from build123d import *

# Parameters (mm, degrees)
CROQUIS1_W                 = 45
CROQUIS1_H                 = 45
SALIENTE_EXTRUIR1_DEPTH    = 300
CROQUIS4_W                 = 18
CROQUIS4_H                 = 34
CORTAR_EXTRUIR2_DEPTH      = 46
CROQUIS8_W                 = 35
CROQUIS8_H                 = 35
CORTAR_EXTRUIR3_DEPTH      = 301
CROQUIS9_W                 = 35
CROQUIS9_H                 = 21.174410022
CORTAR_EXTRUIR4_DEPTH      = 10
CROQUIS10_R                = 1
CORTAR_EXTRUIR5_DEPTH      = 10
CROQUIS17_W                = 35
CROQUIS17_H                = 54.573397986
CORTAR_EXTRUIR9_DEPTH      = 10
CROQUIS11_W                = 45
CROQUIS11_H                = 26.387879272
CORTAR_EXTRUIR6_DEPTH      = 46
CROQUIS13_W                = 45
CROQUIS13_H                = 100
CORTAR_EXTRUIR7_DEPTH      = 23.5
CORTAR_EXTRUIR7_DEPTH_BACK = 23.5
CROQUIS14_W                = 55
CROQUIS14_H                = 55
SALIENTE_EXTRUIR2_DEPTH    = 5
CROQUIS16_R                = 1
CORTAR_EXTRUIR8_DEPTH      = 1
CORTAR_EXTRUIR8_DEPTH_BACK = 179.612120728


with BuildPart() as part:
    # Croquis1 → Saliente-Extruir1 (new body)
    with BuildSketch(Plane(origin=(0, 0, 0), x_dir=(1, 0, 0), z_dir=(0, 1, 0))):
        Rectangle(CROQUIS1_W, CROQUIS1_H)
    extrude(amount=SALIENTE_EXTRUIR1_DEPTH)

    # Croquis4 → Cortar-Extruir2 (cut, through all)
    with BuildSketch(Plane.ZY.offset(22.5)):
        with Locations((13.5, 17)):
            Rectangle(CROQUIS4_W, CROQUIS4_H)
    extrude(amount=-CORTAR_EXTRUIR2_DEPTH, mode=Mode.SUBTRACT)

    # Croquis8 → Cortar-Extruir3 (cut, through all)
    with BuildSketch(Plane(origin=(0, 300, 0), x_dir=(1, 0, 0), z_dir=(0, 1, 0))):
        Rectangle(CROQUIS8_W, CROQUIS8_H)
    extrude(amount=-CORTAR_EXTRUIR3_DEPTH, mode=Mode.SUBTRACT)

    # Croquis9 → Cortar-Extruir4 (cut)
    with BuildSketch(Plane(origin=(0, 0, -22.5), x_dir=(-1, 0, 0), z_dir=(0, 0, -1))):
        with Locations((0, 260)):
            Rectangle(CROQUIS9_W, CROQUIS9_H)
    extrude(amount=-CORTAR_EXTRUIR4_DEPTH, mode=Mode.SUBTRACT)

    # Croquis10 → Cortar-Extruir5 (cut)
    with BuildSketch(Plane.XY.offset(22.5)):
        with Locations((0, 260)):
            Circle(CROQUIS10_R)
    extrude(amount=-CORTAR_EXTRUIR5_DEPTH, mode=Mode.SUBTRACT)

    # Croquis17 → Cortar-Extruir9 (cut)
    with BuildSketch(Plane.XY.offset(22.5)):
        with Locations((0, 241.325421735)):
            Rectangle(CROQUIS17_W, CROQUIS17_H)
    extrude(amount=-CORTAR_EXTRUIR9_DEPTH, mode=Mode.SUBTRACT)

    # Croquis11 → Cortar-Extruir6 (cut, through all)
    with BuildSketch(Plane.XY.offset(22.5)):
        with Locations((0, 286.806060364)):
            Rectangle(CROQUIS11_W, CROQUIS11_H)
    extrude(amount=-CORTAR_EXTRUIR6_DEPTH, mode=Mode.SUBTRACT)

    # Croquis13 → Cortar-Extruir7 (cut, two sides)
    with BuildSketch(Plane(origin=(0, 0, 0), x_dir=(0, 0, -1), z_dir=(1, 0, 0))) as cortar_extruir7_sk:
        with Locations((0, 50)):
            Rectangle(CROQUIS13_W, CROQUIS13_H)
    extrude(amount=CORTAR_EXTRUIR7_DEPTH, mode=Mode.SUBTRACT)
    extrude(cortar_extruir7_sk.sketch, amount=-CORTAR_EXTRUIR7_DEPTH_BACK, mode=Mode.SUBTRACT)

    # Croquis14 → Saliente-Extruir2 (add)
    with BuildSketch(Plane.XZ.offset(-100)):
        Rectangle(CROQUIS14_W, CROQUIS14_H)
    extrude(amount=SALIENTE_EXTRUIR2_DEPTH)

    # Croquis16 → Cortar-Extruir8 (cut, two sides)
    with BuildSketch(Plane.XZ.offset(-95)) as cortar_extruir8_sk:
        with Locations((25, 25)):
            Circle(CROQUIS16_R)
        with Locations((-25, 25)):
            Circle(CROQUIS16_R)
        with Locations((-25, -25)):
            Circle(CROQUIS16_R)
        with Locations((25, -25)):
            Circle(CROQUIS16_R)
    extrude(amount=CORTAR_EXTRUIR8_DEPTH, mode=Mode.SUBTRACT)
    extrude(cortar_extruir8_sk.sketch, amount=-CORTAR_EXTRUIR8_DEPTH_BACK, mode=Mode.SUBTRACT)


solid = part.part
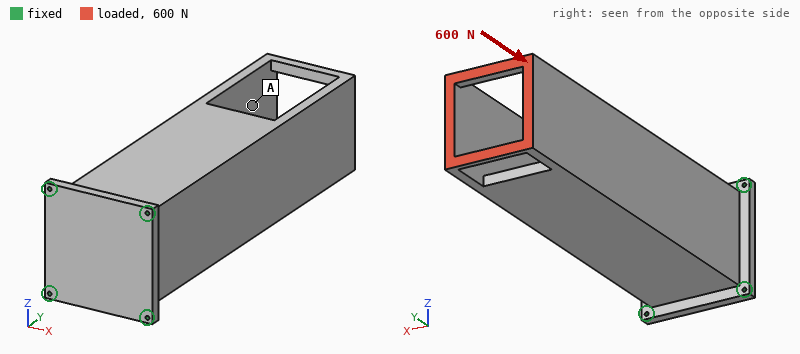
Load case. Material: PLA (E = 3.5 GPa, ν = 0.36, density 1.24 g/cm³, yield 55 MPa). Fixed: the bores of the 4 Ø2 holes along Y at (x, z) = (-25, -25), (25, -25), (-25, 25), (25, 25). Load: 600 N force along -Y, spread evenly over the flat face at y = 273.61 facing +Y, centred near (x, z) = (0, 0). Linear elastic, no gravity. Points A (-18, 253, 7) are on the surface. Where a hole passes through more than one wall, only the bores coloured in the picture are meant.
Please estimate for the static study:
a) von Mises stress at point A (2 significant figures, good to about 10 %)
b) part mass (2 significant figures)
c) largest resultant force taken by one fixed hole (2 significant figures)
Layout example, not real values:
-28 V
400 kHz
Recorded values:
2.7 MPa
170 g
160 N
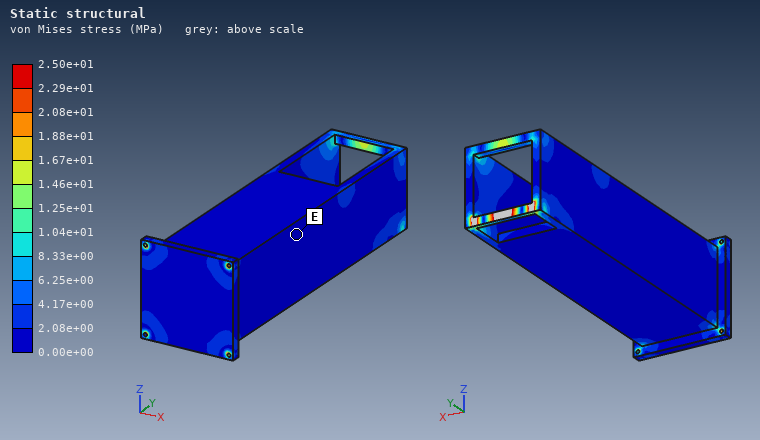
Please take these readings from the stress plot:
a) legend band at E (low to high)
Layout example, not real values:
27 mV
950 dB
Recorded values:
0.00e+00 to 2.08e+00 MPa
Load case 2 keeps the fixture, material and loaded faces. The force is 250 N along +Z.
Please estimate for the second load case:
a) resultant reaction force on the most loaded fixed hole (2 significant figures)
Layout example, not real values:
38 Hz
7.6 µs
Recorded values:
490 N
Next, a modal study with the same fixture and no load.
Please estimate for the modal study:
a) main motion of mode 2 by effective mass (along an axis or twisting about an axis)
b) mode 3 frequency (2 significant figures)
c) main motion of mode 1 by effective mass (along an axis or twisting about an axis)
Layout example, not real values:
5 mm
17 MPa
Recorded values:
along Z
790 Hz
along X
